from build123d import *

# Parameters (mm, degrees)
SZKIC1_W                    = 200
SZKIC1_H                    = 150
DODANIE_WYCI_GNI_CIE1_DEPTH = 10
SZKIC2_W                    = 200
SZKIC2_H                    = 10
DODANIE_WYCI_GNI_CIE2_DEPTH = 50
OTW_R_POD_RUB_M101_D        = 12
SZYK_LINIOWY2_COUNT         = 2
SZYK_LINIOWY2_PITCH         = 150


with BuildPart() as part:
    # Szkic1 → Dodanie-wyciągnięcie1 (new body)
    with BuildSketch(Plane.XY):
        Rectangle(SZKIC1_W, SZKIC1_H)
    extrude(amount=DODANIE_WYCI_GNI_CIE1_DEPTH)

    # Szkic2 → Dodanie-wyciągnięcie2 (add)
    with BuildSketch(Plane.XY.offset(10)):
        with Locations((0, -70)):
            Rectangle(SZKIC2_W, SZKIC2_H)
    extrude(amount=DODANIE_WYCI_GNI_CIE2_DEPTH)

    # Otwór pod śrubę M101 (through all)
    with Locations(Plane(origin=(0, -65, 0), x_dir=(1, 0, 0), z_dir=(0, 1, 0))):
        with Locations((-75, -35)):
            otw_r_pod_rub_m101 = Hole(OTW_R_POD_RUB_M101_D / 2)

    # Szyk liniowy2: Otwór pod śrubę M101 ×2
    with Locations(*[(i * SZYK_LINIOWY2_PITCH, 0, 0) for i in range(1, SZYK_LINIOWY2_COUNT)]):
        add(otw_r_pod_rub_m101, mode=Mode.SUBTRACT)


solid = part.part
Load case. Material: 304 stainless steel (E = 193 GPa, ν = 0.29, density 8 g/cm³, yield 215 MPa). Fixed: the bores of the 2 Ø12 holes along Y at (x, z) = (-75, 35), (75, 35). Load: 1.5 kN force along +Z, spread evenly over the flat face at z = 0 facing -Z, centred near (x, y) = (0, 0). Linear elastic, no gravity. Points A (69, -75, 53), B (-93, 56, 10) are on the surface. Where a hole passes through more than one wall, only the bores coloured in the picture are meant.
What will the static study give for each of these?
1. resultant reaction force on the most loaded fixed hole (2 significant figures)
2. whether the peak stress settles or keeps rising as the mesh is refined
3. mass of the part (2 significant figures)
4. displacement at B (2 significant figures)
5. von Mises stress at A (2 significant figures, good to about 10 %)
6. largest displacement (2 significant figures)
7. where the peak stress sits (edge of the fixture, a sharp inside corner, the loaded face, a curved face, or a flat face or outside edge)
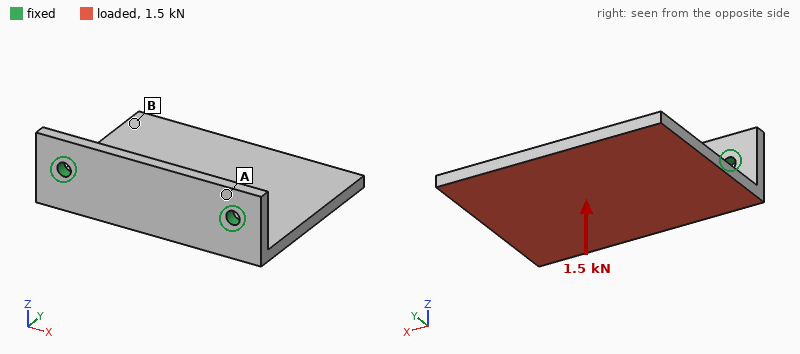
790 N
keeps rising
3.2 kg
0.28 mm
18 MPa
0.33 mm
edge of the fixture
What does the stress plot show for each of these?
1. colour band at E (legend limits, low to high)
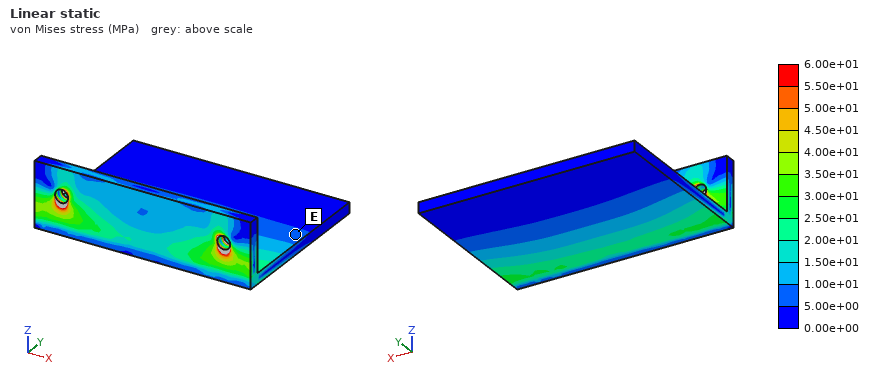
5.00e+00 to 1.00e+01 MPa
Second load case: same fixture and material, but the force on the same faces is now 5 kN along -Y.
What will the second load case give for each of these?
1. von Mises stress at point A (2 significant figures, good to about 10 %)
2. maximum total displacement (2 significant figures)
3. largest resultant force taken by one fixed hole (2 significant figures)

14 MPa
0.23 mm
2.5 kN
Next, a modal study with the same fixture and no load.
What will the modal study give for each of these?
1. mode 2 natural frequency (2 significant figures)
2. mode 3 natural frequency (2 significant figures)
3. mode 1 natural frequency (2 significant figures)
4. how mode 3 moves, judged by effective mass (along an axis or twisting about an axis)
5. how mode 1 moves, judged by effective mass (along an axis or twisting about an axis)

640 Hz
1400 Hz
270 Hz
along X
along Z
